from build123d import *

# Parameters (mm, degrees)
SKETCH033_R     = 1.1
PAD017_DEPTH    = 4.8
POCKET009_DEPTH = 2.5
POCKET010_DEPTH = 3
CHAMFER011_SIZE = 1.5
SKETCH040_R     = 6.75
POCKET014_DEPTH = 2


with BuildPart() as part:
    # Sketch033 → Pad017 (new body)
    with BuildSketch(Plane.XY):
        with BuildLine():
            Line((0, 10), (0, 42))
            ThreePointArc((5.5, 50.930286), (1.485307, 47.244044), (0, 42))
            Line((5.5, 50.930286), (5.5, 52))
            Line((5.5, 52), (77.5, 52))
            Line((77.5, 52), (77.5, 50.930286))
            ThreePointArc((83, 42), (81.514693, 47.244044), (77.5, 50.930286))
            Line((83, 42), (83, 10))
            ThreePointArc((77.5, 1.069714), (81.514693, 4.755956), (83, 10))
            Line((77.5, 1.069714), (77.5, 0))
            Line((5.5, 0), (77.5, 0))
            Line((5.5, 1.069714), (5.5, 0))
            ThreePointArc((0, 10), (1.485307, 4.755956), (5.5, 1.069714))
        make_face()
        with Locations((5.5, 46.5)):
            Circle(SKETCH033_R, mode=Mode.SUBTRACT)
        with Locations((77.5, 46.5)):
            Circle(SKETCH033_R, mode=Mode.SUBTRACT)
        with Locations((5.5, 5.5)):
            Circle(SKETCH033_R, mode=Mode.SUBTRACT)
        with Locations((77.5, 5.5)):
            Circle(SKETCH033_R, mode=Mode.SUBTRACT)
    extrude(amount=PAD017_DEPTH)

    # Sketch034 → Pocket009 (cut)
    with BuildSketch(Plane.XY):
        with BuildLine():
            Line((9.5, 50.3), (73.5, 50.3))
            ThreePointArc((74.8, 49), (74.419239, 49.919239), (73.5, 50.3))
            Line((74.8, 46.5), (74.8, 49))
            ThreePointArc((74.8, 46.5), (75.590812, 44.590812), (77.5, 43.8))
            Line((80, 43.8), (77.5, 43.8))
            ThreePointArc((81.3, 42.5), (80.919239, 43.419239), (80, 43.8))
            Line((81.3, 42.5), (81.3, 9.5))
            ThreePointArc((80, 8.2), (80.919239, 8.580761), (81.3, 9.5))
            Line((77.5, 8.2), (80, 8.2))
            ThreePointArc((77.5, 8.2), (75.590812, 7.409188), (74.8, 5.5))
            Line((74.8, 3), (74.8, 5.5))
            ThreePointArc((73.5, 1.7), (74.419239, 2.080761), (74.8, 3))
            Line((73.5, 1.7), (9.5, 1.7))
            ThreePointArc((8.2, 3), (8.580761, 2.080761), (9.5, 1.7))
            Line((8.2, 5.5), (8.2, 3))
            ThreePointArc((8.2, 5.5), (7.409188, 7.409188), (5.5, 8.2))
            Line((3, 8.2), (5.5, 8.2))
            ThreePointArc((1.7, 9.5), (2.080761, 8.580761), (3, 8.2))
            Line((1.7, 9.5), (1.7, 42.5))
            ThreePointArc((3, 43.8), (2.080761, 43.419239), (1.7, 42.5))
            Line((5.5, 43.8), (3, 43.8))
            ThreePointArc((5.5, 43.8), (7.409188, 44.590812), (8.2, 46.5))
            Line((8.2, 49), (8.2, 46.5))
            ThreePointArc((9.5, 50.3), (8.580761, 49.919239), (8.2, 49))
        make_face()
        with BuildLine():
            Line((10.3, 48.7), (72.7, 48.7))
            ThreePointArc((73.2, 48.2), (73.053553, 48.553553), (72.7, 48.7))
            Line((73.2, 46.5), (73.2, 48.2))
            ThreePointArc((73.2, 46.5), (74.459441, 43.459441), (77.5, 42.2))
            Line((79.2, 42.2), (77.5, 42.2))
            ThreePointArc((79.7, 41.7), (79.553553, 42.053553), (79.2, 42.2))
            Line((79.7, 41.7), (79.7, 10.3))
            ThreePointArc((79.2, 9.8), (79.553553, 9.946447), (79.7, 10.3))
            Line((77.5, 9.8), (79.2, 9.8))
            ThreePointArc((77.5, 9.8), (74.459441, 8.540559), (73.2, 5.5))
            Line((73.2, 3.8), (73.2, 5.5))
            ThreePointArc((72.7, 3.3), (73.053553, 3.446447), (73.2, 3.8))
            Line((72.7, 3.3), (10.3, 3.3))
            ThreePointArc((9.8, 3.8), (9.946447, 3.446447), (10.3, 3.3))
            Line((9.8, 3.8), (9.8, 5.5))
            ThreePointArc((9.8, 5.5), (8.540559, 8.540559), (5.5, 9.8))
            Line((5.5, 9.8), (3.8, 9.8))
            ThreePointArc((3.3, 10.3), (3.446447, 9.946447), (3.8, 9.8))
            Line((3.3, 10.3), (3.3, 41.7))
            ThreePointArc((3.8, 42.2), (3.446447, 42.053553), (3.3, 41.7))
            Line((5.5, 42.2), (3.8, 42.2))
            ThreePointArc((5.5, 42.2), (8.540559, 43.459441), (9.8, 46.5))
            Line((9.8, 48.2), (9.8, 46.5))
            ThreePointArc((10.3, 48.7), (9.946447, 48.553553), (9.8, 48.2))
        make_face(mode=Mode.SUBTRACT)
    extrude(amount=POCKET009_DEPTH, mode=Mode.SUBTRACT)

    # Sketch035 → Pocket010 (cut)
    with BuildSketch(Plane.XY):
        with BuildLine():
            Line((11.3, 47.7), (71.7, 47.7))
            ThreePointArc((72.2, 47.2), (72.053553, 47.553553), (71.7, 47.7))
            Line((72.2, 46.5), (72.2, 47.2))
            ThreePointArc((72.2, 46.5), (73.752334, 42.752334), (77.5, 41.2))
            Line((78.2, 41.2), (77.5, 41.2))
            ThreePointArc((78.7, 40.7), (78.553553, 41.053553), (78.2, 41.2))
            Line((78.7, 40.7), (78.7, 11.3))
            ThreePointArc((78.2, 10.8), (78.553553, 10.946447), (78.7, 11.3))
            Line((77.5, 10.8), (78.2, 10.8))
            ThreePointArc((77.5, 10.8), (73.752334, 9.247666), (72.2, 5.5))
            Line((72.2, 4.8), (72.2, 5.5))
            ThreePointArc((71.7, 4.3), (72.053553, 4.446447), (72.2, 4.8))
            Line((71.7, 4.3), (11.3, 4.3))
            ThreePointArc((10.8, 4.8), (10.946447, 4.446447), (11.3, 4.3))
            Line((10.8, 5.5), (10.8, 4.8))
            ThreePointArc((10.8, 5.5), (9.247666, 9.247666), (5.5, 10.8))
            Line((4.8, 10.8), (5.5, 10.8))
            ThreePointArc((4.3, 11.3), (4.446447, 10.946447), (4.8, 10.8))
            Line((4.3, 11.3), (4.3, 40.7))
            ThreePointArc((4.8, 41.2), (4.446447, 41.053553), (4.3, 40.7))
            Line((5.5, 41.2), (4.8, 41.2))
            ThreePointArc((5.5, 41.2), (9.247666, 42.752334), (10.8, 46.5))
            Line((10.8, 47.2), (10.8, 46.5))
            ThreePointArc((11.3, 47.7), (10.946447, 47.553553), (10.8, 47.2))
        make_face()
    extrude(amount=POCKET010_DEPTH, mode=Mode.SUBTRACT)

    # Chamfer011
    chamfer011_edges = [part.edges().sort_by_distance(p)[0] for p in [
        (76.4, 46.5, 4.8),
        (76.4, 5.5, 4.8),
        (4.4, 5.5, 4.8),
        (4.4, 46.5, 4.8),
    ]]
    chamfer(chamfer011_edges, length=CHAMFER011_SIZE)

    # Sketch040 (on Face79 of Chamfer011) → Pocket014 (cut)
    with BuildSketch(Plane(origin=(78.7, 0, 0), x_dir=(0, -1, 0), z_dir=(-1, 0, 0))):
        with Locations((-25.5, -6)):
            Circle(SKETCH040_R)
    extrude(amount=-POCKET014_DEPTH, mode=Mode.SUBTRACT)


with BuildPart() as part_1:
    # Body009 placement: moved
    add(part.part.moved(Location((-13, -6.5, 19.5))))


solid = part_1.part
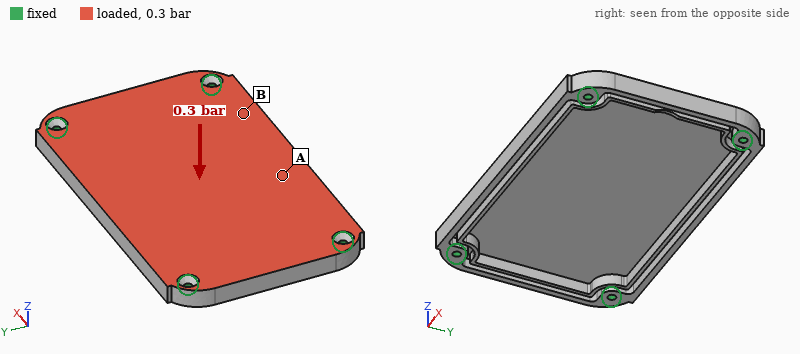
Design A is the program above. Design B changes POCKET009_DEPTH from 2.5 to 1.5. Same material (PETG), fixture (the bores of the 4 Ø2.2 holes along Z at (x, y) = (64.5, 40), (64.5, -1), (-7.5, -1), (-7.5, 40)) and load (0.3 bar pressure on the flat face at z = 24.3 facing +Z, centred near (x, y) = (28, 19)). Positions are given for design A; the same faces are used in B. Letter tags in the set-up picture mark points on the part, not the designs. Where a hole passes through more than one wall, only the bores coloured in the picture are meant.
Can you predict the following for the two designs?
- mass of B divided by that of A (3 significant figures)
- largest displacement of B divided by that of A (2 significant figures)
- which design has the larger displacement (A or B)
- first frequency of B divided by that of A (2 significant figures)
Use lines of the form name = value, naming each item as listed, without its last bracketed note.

mass of B divided by that of A = 1.04
largest displacement of B divided by that of A = 0.84
which design has the larger displacement = A
first frequency of B divided by that of A = 1.1
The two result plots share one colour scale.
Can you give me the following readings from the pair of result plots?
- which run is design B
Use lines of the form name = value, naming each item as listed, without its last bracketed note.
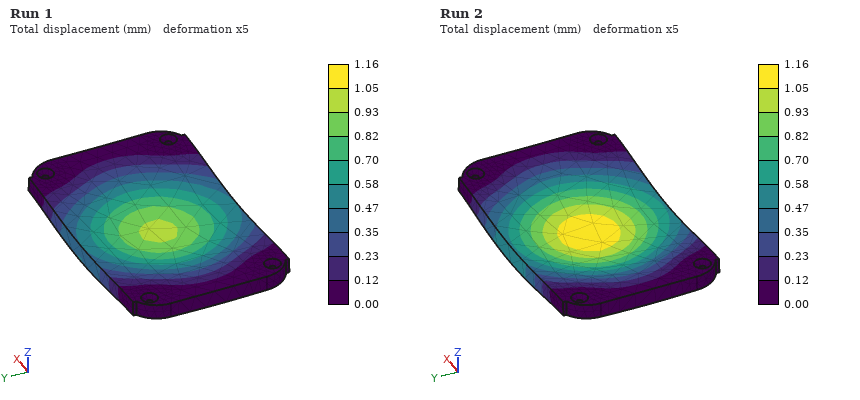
which run is design B = Run 1
